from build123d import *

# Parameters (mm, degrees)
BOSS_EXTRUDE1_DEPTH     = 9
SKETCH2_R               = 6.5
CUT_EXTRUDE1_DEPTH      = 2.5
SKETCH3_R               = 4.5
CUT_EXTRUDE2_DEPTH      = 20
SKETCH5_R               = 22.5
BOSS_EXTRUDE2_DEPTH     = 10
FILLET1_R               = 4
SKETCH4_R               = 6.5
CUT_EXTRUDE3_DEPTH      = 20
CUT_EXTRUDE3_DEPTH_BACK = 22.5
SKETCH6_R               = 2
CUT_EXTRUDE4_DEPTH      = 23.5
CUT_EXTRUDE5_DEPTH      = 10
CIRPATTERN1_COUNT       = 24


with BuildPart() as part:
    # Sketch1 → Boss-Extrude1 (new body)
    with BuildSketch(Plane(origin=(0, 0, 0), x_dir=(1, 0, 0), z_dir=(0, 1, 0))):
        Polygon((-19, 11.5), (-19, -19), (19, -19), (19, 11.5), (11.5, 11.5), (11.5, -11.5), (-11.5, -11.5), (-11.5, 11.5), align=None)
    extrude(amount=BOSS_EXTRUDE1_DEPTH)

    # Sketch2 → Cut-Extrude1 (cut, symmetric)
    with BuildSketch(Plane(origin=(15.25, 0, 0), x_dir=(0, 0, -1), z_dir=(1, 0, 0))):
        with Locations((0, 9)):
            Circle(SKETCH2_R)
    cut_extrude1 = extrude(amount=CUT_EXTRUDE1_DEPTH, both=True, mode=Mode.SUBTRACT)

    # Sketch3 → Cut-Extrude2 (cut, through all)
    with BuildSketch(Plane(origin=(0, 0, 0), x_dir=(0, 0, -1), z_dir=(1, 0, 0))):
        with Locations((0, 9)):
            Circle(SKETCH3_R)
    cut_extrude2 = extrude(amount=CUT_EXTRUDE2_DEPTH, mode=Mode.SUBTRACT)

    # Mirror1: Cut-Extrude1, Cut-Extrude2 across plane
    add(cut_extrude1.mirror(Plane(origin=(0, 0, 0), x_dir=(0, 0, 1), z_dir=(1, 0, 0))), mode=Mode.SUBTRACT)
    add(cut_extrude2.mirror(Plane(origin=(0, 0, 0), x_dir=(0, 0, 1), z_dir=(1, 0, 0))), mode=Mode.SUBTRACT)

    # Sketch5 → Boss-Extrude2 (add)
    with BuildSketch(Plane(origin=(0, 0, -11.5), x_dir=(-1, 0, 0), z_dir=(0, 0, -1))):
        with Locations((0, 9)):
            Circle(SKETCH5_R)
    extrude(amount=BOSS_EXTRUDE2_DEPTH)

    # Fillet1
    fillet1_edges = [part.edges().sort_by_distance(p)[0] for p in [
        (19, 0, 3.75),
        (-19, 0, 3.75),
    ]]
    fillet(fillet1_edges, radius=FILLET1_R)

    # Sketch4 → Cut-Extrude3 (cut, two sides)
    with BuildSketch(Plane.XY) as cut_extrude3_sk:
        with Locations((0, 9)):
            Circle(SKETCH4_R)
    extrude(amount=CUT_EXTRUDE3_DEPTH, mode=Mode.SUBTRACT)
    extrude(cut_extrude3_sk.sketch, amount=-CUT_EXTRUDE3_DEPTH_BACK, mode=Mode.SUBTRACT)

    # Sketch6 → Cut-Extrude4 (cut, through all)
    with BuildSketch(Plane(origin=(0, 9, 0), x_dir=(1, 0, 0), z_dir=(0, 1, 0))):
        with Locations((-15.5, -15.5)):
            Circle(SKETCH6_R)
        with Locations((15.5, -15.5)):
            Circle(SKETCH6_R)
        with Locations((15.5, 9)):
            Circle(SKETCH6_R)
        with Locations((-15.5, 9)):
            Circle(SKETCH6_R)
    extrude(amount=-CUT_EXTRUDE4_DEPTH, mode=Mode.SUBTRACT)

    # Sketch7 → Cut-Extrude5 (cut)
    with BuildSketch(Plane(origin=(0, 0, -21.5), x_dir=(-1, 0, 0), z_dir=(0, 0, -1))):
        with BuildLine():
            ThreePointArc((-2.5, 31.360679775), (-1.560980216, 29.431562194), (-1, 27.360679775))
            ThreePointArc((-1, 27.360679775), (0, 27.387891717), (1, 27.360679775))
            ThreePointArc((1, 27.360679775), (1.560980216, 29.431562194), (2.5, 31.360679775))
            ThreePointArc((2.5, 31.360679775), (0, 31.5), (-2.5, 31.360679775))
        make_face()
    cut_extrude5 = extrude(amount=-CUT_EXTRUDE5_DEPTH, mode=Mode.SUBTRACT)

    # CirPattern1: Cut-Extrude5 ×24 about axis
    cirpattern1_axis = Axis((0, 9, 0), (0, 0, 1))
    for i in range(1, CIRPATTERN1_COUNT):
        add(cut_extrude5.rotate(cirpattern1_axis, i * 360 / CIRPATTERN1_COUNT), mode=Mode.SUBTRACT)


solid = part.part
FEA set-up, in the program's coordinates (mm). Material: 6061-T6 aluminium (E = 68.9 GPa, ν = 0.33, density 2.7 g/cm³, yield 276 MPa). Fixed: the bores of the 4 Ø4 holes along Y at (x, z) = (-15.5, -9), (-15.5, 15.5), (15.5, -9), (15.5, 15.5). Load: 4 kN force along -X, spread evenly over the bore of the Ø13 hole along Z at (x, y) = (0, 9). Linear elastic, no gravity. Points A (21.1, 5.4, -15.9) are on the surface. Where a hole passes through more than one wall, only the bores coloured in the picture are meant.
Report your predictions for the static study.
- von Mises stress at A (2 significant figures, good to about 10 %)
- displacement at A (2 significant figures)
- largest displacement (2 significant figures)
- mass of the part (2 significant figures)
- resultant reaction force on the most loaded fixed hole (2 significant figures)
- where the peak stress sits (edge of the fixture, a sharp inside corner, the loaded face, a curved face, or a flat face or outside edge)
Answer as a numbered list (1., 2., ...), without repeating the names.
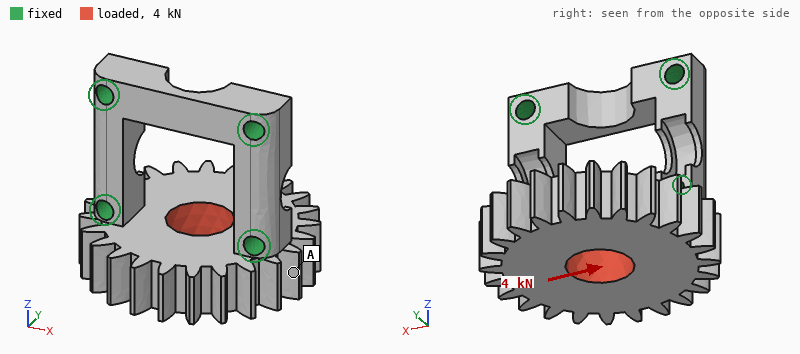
1. 9.9 MPa
2. 7.5 µm
3. 13 µm
4. 41 g
5. 2.2 kN
6. edge of the fixture
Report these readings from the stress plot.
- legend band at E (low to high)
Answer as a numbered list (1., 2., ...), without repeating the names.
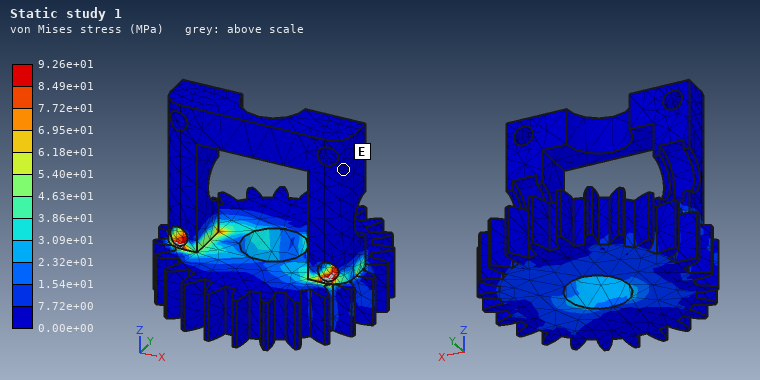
1. 0.00e+00 to 7.72e+00 MPa
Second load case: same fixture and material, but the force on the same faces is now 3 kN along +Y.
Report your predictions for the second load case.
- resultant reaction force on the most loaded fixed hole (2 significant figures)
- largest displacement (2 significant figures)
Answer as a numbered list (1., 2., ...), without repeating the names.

1. 1.5 kN
2. 37 µm
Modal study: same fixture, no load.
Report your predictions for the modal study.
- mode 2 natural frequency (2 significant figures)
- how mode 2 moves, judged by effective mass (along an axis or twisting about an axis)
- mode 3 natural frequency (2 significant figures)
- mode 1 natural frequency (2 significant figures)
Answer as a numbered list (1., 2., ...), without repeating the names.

1. 16 kHz
2. along X
3. 18 kHz
4. 7200 Hz
